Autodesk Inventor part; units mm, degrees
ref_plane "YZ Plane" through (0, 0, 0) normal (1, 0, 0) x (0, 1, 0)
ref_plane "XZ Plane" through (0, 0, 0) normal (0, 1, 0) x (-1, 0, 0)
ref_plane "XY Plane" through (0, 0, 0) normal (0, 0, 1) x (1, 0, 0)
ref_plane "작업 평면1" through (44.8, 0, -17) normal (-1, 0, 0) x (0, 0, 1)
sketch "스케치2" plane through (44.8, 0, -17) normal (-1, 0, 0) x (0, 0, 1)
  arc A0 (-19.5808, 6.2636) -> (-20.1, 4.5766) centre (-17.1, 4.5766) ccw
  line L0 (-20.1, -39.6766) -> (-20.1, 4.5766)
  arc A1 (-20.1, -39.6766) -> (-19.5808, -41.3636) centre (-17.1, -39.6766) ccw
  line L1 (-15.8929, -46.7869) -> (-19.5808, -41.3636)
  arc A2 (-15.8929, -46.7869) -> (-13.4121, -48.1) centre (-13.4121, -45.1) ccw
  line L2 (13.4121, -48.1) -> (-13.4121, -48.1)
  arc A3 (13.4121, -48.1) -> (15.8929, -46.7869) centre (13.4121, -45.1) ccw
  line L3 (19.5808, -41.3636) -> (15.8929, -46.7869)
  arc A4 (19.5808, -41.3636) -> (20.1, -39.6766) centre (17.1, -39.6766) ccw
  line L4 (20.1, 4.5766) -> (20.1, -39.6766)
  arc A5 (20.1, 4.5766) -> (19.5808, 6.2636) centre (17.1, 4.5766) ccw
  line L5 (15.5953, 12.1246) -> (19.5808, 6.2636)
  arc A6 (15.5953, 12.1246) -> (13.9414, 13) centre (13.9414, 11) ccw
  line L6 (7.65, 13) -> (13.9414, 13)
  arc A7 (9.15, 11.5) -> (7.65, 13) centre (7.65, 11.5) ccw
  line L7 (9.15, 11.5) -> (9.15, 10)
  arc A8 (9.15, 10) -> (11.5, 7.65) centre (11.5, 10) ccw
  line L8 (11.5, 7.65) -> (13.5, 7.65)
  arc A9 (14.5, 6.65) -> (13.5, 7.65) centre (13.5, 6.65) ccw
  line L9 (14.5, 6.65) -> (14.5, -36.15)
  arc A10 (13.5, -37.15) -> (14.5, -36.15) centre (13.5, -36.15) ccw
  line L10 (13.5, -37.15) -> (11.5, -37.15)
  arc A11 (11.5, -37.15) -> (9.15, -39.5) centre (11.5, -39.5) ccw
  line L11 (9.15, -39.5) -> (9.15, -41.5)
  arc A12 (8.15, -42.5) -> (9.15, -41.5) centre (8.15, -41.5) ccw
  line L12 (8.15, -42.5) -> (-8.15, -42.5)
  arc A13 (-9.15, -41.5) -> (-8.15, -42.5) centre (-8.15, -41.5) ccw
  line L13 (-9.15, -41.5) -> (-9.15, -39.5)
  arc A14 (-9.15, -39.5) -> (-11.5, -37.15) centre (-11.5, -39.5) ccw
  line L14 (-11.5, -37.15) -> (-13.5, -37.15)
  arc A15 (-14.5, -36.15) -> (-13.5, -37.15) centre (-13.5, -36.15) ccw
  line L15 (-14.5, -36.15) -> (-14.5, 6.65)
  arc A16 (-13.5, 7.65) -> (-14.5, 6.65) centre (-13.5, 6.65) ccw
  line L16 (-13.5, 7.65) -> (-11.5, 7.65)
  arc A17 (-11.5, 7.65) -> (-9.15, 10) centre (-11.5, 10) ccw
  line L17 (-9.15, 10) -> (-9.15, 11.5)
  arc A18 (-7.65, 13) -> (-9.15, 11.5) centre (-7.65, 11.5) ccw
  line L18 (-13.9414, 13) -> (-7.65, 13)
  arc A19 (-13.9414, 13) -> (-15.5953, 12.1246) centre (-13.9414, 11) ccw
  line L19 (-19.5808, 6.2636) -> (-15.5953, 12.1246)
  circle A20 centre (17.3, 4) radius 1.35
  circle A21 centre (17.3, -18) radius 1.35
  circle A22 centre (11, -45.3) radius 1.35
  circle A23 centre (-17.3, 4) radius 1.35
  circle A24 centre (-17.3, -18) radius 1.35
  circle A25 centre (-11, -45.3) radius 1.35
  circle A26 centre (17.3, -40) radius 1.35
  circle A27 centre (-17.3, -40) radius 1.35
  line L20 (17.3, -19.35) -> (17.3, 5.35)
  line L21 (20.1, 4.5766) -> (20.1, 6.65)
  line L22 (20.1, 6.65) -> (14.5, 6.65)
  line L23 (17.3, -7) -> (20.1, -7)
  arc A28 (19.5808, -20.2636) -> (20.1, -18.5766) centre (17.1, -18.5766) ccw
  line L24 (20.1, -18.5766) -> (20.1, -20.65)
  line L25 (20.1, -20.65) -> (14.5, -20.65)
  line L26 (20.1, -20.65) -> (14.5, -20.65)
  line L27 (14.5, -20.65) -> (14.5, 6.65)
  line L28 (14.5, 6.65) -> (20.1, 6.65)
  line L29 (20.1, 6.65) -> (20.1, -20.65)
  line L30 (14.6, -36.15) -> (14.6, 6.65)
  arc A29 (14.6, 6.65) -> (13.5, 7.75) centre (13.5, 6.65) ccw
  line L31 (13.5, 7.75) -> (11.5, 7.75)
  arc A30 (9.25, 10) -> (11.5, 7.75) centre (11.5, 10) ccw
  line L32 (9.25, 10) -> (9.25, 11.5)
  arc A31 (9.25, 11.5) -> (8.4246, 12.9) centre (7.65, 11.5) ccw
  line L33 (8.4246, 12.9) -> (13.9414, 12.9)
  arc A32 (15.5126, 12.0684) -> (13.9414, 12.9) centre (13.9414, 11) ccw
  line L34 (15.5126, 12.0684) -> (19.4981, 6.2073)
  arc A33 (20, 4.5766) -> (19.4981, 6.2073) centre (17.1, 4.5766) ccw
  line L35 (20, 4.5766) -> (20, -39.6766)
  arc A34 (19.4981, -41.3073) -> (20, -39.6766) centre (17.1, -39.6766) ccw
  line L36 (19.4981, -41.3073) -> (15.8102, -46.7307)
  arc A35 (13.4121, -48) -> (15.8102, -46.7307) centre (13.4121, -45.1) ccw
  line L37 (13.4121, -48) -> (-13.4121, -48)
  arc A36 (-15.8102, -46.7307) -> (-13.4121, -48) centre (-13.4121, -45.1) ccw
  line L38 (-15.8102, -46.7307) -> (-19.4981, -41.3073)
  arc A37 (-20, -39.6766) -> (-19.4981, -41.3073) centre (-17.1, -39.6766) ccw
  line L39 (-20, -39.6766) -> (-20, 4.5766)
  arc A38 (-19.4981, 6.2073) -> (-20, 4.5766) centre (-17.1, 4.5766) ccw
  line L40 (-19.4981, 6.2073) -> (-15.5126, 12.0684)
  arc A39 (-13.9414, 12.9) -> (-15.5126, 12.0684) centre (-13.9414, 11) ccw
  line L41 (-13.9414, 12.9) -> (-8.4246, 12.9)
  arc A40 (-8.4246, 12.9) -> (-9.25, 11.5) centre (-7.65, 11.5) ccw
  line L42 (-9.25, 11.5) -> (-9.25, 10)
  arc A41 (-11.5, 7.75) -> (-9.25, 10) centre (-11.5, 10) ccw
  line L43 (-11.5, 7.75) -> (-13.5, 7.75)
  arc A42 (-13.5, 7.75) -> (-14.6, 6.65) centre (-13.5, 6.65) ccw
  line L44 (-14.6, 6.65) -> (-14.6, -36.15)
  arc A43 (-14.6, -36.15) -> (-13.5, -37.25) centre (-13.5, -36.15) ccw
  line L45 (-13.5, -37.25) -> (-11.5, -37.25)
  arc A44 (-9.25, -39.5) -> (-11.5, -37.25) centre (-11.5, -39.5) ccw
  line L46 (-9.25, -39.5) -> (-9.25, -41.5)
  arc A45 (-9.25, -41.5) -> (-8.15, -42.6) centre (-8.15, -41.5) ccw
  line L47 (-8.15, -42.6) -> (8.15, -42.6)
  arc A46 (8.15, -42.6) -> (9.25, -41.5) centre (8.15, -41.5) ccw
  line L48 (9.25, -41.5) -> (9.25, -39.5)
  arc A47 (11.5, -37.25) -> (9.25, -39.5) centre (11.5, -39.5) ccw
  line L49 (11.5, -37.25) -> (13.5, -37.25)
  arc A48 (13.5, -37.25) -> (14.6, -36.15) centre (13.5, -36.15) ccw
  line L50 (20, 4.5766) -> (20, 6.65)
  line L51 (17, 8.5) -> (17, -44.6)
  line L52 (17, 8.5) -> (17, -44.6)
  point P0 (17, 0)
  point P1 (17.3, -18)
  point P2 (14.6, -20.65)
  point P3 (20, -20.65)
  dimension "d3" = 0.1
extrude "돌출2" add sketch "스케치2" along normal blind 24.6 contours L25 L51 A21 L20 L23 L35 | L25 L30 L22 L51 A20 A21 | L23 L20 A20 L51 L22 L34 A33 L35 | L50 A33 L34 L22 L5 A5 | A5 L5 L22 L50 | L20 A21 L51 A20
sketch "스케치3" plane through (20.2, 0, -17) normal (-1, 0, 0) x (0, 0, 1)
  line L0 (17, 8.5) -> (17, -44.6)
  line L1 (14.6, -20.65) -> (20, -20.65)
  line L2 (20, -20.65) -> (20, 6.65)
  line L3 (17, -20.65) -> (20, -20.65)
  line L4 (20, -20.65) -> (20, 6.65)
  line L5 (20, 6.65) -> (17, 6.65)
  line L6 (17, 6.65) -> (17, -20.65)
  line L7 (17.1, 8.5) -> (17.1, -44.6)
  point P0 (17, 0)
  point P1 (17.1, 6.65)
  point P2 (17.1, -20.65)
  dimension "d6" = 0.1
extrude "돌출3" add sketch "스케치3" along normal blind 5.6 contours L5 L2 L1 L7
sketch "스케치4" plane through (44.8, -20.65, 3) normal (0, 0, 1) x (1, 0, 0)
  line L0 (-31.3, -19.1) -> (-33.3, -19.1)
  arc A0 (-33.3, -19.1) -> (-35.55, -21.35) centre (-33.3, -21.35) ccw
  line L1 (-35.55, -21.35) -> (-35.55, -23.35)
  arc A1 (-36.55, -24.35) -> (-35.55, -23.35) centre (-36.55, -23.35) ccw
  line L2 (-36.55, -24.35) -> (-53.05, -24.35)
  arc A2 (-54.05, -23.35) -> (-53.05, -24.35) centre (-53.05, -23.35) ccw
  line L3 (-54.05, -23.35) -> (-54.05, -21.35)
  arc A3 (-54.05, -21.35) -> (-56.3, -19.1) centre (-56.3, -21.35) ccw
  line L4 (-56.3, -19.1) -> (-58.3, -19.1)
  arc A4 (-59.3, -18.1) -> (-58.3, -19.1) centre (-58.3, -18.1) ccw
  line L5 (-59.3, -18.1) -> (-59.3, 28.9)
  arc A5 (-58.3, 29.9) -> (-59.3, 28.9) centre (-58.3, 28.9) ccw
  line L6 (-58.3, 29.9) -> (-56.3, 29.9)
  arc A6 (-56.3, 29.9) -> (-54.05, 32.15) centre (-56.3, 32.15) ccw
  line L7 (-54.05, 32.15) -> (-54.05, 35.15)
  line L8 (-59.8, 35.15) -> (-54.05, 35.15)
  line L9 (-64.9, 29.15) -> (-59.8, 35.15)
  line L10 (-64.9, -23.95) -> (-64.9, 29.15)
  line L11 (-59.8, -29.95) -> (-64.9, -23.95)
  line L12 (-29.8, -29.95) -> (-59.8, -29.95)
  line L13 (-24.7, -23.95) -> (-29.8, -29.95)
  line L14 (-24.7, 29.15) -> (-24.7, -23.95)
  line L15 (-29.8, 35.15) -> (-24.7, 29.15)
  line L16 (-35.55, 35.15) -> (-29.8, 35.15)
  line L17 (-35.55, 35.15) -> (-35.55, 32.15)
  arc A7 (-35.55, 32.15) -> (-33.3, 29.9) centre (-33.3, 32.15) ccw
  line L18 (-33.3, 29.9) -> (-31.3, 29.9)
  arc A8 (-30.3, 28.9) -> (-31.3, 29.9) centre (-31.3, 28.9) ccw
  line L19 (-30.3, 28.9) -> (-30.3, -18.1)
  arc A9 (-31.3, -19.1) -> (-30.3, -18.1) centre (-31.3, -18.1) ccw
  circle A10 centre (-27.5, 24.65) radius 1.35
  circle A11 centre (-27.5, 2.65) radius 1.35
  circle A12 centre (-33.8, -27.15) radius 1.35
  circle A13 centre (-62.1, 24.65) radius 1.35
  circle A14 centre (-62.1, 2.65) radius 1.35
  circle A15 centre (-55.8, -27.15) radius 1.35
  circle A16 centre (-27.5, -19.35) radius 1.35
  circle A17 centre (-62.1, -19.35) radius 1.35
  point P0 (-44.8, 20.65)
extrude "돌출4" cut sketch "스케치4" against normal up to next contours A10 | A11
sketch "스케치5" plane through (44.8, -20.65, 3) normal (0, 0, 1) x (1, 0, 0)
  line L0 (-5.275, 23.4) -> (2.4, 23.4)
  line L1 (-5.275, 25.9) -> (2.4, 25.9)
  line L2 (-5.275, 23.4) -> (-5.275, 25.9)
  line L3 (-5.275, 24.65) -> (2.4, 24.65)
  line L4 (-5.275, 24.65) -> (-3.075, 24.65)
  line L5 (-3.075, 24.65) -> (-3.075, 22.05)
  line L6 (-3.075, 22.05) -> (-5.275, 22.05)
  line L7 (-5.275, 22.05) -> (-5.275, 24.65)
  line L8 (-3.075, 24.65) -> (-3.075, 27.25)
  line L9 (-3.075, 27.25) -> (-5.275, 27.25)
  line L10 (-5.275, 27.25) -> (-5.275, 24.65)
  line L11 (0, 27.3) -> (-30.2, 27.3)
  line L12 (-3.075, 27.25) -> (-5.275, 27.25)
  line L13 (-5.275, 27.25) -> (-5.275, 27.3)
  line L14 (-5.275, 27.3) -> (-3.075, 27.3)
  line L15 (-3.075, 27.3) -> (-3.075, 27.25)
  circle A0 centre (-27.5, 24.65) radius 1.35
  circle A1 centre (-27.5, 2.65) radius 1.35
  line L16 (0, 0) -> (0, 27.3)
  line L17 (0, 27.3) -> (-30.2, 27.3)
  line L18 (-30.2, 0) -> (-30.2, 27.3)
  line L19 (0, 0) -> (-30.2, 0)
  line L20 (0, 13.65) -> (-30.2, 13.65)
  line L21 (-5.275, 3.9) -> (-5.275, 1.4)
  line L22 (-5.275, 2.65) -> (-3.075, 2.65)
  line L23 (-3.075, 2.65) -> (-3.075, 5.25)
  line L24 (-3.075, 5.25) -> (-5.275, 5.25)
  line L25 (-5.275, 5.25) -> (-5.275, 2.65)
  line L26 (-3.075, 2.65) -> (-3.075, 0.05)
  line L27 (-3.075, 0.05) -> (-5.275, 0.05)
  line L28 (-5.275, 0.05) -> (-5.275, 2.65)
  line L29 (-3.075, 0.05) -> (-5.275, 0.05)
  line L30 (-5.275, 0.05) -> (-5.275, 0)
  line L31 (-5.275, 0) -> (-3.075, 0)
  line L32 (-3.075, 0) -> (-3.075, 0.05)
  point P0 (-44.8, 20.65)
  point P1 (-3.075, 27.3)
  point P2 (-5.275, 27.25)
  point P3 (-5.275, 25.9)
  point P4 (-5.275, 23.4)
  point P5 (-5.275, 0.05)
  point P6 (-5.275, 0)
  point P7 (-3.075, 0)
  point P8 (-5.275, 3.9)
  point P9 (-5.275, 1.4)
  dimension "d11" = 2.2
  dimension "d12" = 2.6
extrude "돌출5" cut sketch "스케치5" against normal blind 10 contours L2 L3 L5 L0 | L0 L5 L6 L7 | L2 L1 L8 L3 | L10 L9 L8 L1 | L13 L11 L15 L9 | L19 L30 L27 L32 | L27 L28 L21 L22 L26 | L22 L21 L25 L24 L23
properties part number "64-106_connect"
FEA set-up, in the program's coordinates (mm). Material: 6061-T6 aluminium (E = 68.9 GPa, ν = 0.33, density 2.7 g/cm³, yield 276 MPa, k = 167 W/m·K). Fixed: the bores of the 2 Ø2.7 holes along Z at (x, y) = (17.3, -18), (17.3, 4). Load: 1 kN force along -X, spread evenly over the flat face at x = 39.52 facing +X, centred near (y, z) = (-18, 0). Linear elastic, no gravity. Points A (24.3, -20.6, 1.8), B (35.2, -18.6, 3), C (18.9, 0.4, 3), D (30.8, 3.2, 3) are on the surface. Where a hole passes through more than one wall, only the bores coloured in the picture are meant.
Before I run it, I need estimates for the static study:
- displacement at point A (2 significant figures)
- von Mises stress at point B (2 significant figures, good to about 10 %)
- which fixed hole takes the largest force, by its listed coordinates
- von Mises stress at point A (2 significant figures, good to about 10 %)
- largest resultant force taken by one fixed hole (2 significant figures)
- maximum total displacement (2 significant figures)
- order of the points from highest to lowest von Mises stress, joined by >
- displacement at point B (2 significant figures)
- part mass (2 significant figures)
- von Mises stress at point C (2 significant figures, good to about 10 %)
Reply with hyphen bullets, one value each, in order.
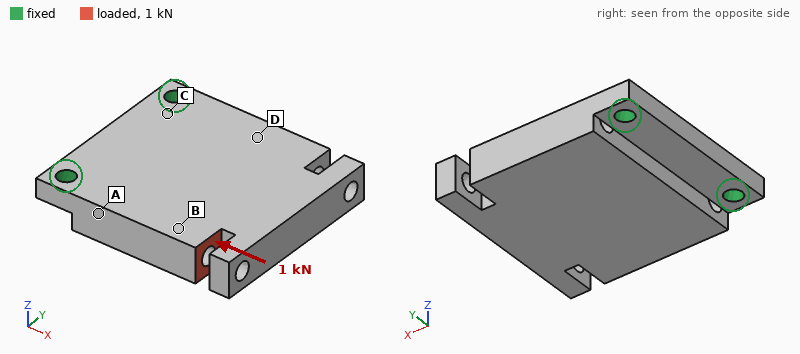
- 14 µm
- 38 MPa
- (17.3, -18)
- 51 MPa
- 1.0 kN
- 67 µm
- A > B > C > D
- 41 µm
- 9.9 g
- 22 MPa
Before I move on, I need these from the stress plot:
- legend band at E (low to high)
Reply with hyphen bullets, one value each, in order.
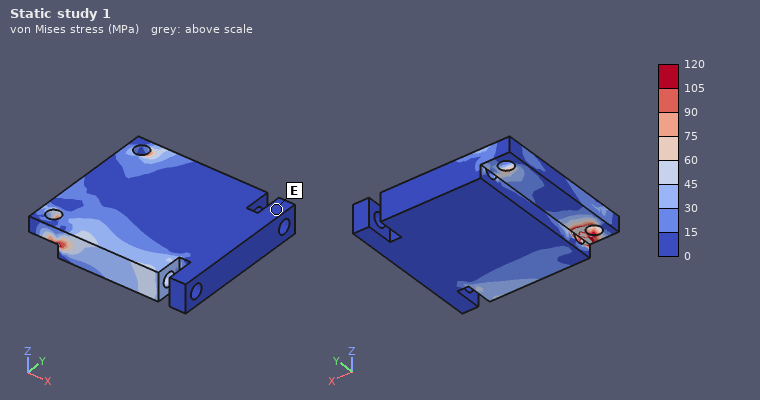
- 0 to 15 MPa
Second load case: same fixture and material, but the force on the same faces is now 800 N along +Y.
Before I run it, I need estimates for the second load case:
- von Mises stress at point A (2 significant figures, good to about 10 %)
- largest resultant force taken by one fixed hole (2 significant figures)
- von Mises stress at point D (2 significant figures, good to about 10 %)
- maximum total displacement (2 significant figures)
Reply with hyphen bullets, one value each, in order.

- 35 MPa
- 890 N
- 18 MPa
- 31 µm
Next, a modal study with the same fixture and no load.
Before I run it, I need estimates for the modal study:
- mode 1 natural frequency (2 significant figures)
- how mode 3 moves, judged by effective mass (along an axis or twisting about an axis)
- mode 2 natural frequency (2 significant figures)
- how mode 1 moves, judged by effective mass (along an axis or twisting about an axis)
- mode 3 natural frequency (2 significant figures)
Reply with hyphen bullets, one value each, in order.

- 2600 Hz
- along Y
- 12 kHz
- along Z
- 16 kHz
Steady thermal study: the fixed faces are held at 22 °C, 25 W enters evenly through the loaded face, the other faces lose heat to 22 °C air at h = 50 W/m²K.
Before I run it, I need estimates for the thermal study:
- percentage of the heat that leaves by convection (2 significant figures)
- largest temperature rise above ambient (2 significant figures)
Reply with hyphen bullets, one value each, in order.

- 11 %
- 62 K
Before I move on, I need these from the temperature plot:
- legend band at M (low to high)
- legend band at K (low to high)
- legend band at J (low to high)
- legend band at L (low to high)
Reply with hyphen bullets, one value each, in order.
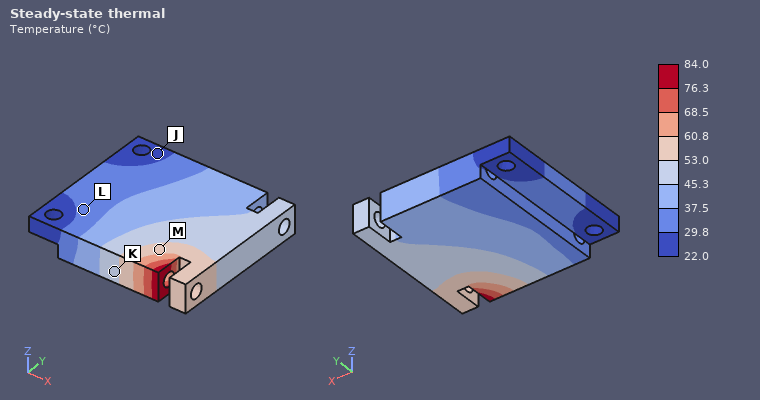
- 53.0 to 60.8 °C
- 45.3 to 53.0 °C
- 22.0 to 29.8 °C
- 29.8 to 37.5 °C
